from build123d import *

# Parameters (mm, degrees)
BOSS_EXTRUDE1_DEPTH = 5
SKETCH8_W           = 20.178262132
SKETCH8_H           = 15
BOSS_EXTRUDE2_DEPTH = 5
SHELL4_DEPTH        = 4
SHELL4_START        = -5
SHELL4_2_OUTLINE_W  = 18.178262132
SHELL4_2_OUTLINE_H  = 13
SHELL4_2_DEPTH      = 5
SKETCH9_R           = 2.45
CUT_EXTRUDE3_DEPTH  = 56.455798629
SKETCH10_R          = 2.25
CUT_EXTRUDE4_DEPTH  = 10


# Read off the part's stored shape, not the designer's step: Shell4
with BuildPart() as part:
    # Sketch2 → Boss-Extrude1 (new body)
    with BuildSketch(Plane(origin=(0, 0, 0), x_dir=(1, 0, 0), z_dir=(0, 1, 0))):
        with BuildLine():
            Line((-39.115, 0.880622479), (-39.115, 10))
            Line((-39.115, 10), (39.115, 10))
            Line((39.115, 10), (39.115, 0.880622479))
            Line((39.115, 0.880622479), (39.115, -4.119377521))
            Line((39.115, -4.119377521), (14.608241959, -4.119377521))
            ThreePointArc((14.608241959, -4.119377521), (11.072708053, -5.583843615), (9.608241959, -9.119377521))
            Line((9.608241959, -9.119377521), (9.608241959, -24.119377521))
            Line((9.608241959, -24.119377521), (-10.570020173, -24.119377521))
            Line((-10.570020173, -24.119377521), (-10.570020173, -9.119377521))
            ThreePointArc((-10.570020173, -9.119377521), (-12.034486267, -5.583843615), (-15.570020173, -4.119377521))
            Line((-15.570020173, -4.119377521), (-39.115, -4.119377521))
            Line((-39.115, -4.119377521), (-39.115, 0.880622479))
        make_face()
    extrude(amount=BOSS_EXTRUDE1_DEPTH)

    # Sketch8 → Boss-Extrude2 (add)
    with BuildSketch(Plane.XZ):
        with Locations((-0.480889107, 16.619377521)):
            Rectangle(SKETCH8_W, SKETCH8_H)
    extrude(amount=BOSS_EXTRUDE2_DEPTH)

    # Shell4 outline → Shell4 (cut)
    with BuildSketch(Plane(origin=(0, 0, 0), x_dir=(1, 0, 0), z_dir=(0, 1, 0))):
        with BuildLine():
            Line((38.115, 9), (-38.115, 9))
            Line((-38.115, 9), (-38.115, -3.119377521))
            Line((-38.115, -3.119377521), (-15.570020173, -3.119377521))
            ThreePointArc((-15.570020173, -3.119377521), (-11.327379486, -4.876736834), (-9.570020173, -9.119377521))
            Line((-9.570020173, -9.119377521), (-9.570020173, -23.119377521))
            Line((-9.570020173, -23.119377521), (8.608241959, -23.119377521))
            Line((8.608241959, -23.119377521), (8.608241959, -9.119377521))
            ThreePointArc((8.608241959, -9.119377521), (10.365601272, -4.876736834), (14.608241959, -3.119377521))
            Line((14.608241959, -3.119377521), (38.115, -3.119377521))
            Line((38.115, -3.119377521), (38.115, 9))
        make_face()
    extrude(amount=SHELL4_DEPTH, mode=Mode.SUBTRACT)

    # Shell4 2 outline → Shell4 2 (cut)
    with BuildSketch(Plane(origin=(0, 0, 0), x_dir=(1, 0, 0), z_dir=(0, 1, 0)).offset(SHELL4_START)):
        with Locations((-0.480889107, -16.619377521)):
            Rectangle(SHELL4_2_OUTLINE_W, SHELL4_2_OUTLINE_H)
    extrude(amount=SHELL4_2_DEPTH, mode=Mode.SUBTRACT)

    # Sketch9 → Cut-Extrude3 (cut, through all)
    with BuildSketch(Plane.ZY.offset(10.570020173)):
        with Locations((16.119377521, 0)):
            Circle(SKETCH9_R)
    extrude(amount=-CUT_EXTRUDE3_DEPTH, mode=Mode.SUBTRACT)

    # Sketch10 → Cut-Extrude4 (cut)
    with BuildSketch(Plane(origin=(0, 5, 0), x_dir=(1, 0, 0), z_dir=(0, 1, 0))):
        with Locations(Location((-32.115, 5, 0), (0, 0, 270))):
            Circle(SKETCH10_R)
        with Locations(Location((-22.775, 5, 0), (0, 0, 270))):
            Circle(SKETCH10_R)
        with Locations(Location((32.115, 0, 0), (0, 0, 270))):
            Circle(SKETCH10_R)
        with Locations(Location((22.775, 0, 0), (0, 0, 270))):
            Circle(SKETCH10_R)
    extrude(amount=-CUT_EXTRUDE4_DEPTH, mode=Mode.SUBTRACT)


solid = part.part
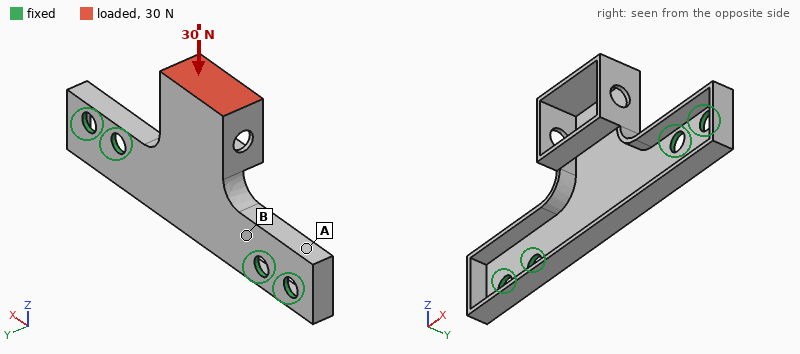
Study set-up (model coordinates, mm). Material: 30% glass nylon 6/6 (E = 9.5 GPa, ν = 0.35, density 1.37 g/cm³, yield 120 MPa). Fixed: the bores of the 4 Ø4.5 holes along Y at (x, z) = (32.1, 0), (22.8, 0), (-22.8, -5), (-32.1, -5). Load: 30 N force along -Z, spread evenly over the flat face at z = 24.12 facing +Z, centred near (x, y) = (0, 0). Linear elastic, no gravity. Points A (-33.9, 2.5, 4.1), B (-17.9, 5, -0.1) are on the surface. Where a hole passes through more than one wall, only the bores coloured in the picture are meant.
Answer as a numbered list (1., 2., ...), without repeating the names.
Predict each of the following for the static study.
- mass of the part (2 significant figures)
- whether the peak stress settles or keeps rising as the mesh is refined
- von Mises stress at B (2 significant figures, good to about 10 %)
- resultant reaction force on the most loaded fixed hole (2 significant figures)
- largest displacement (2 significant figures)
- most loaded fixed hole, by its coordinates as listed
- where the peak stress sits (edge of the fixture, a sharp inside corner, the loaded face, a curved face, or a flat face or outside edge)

1. 3.6 g
2. keeps rising
3. 9.5 MPa
4. 24 N
5. 0.99 mm
6. (-22.8, -5)
7. edge of the fixture
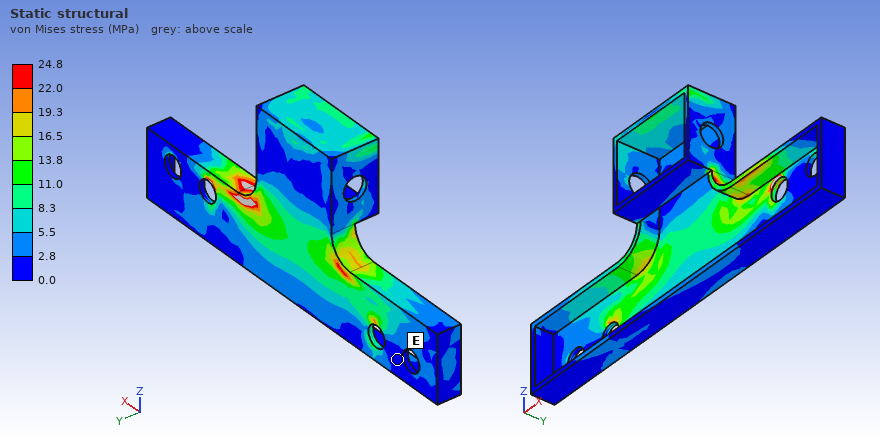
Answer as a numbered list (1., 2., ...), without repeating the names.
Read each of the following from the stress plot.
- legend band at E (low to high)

1. 0.0 to 2.8 MPa
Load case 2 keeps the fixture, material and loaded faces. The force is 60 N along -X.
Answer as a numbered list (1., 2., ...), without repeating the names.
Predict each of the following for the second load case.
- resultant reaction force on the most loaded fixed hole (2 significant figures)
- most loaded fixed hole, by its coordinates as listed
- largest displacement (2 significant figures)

1. 55 N
2. (22.8, 0)
3. 0.96 mm
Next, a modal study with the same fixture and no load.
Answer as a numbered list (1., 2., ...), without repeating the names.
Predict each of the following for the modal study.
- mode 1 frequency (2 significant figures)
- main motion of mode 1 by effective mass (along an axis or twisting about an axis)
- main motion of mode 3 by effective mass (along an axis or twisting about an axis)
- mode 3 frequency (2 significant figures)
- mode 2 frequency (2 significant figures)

1. 510 Hz
2. along Y
3. along Y
4. 2800 Hz
5. 1600 Hz
